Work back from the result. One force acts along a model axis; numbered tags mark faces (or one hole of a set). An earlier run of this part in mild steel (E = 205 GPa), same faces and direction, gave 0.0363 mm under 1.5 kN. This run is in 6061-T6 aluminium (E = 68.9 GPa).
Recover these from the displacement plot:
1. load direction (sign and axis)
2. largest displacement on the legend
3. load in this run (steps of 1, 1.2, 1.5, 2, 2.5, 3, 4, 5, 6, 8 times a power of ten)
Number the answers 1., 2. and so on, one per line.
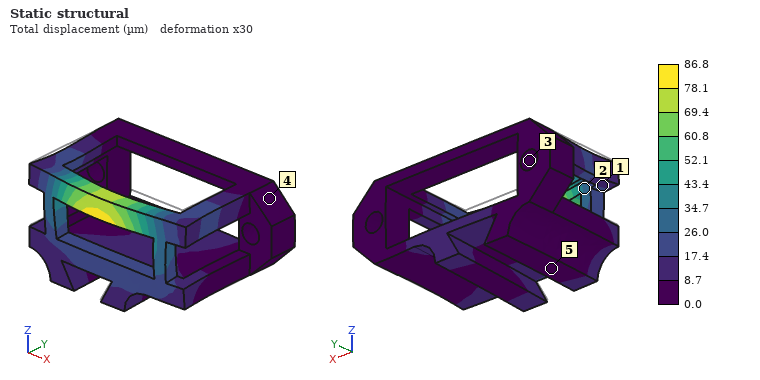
1. -Y
2. 86.8 µm
3. 1.2 kN
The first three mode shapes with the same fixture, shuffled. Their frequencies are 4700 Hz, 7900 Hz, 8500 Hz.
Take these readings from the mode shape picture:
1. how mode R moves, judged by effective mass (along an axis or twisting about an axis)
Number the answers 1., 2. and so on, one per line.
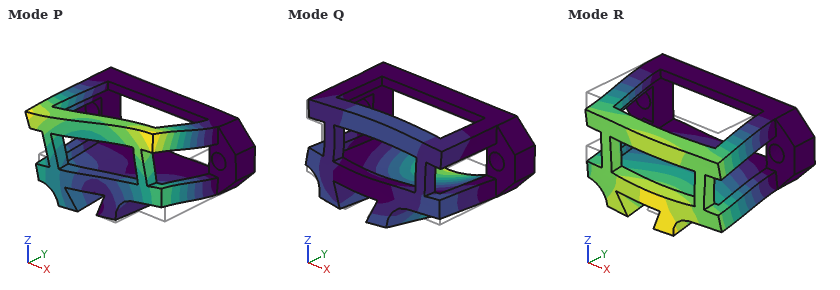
1. along Z
